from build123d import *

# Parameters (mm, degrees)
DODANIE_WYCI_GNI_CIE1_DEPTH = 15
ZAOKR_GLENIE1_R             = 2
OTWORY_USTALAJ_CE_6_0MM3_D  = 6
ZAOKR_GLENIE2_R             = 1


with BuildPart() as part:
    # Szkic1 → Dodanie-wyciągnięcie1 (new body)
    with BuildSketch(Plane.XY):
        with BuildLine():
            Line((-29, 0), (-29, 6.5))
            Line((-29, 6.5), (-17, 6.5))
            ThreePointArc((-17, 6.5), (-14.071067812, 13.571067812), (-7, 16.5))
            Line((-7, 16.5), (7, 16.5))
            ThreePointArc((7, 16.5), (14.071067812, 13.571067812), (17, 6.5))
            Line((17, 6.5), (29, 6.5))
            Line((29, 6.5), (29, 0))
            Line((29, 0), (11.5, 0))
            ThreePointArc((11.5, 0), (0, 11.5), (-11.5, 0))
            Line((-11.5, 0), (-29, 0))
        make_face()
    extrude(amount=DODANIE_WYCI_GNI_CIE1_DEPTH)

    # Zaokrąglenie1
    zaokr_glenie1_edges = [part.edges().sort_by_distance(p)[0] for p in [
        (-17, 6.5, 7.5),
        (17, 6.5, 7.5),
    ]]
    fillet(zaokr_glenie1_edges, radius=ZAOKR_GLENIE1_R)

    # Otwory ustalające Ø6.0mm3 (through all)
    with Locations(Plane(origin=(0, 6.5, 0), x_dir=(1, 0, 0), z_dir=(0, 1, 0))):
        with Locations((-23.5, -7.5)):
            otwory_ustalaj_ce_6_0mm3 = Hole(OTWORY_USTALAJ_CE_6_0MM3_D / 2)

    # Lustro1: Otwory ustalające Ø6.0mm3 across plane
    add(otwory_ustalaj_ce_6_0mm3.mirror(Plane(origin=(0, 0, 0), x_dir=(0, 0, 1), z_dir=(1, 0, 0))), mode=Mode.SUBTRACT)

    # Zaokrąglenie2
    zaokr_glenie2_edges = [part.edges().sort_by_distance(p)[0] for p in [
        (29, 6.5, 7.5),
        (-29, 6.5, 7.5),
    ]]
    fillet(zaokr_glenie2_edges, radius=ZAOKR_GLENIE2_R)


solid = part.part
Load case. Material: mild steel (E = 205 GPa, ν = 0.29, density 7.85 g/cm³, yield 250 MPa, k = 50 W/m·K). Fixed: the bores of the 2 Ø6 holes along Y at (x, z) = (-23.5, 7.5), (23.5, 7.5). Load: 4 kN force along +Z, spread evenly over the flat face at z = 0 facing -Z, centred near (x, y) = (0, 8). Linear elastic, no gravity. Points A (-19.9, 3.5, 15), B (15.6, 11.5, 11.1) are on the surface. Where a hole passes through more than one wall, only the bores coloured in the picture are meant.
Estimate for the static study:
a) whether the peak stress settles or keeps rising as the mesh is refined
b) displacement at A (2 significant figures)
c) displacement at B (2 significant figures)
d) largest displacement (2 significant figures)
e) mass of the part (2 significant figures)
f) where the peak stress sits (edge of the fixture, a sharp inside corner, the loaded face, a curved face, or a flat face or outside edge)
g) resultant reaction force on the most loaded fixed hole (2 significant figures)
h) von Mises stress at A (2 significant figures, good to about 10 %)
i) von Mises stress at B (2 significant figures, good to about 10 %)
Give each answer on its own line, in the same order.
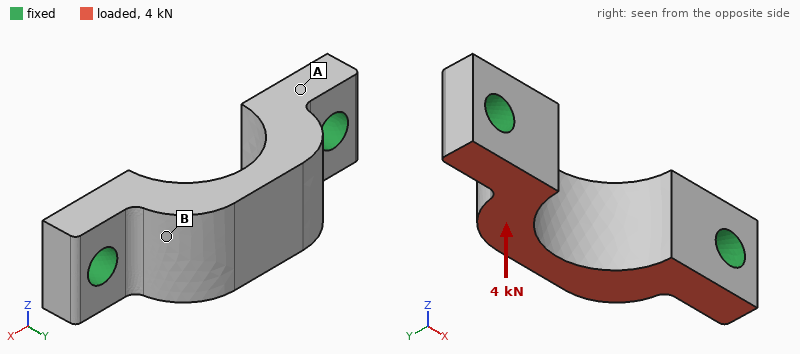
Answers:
keeps rising
2.9 µm
8.3 µm
16 µm
52 g
edge of the fixture
2.0 kN
64 MPa
27 MPa
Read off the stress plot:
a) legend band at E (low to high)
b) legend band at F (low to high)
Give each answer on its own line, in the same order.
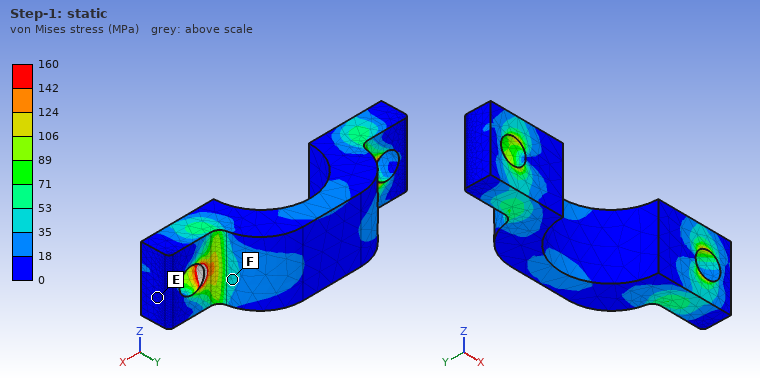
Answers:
0 to 18 MPa
35 to 53 MPa
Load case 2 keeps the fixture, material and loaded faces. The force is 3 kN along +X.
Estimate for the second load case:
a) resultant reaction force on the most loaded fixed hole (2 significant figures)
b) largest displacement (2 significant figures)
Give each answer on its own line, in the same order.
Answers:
1.6 kN
4.0 µm
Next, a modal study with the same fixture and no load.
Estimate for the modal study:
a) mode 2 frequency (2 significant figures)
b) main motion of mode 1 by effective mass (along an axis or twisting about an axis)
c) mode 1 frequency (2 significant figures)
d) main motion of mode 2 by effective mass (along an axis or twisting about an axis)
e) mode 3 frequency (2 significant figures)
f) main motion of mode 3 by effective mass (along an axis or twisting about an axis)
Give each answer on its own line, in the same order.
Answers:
24 kHz
along Z
13 kHz
along Y
26 kHz
along X
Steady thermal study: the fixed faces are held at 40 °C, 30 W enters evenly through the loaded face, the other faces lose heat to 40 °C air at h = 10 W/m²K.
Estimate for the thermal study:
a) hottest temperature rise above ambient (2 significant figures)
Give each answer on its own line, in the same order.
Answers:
35 K
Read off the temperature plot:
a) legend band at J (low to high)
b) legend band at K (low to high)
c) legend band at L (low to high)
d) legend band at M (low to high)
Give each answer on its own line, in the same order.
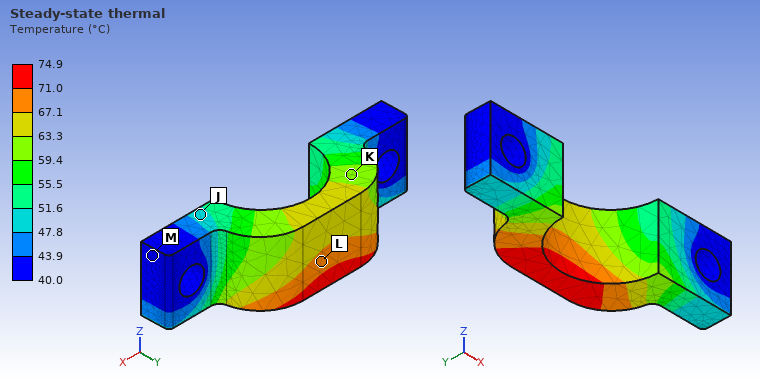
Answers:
47.8 to 51.6 °C
59.4 to 63.3 °C
67.1 to 71.0 °C
40.0 to 43.9 °C
